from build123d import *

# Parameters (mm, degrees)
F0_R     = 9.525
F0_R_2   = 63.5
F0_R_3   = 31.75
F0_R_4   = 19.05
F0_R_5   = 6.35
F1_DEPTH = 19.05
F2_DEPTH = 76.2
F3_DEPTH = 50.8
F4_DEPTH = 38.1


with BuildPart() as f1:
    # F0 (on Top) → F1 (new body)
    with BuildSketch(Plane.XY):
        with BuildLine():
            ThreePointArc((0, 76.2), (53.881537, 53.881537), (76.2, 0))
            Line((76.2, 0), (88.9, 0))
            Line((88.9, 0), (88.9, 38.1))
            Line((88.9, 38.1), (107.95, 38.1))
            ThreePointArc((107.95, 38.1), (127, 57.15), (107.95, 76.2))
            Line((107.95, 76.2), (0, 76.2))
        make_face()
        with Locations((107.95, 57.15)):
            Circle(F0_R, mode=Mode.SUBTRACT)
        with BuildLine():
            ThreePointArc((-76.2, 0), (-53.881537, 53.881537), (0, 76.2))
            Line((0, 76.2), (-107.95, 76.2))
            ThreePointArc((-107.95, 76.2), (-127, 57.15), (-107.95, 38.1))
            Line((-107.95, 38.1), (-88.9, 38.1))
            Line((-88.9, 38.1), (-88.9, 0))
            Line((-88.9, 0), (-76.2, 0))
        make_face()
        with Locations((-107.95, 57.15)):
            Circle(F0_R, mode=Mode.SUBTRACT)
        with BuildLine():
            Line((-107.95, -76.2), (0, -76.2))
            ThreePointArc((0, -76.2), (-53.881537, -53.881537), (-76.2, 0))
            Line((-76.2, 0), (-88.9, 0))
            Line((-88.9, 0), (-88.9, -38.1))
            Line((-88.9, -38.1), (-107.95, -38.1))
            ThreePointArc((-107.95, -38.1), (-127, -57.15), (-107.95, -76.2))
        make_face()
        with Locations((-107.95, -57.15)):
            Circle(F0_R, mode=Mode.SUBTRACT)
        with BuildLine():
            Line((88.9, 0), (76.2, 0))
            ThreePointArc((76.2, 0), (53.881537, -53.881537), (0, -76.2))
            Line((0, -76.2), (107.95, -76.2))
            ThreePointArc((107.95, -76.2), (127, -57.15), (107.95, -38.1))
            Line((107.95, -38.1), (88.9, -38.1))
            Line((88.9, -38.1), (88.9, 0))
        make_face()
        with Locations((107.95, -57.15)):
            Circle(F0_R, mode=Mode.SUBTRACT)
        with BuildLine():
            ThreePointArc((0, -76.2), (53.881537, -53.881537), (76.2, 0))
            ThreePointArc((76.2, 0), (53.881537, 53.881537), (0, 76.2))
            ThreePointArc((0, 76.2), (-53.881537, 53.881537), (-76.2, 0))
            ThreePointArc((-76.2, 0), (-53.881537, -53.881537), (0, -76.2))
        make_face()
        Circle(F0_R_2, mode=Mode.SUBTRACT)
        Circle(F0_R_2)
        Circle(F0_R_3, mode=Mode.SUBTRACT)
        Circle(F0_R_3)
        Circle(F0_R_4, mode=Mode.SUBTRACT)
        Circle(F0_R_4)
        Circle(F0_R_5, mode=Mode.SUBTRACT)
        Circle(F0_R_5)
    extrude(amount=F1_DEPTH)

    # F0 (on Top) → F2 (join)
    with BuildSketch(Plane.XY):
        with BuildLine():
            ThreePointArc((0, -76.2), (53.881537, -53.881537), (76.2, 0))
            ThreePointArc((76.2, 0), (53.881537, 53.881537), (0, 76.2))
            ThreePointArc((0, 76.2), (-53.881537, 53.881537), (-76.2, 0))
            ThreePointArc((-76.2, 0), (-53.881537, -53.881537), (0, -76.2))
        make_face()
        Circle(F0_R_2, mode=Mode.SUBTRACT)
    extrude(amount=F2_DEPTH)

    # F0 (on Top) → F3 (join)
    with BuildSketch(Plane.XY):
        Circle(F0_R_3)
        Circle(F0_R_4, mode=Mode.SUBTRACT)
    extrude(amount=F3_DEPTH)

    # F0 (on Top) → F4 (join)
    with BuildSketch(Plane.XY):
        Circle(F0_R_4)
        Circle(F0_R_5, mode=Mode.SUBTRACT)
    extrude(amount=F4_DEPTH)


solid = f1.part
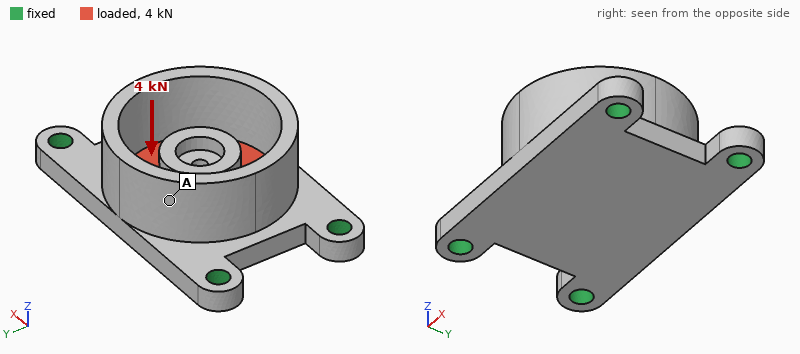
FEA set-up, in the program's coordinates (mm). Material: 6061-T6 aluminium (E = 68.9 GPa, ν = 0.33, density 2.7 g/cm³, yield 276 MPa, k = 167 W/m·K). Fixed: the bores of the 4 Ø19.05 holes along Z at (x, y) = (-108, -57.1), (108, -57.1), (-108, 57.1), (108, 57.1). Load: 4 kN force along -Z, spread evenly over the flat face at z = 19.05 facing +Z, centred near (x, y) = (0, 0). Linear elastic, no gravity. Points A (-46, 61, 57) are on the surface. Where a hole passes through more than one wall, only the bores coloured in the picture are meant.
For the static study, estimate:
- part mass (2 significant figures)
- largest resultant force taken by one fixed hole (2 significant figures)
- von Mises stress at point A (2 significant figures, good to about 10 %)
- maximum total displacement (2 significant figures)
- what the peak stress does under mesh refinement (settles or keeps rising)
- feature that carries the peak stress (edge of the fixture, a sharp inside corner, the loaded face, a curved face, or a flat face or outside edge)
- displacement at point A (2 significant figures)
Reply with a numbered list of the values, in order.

1. 2.7 kg
2. 1.1 kN
3. 1.9 MPa
4. 18 µm
5. keeps rising
6. edge of the fixture
7. 14 µm
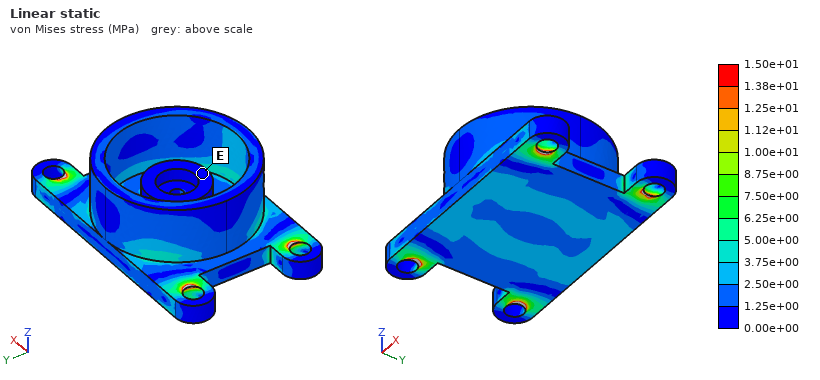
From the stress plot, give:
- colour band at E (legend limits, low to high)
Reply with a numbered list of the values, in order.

1. 0.00e+00 to 1.25e+00 MPa
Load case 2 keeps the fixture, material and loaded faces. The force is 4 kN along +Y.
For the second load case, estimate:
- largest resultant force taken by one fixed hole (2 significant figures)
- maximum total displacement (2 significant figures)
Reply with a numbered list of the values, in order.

1. 1.2 kN
2. 6.0 µm
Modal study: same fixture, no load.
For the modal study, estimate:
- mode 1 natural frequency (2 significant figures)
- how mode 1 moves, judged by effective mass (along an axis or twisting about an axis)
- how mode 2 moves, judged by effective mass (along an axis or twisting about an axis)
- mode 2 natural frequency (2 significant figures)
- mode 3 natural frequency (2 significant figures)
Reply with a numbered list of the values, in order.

1. 1800 Hz
2. along Z
3. along Y
4. 2100 Hz
5. 3400 Hz
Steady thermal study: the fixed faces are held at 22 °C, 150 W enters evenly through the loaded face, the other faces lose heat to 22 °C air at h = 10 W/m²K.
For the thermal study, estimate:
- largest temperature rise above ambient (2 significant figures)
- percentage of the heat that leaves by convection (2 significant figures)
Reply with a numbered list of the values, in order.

1. 15 K
2. 8.8 %
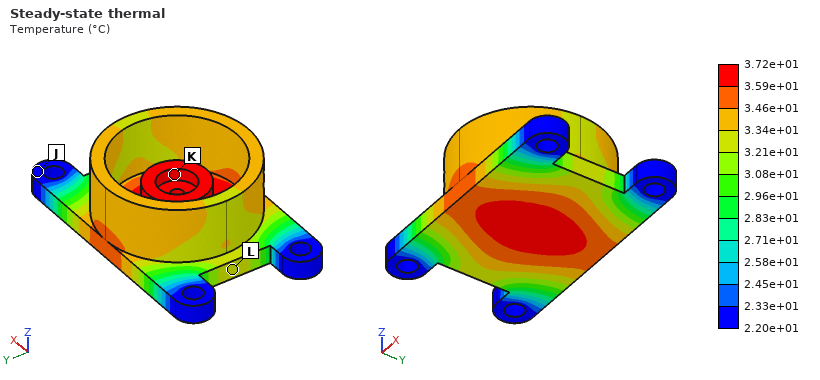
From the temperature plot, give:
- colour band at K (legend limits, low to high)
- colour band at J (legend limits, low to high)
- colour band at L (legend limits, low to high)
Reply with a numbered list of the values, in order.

1. 3.59e+01 to 3.72e+01 °C
2. 2.20e+01 to 2.33e+01 °C
3. 3.21e+01 to 3.34e+01 °C
